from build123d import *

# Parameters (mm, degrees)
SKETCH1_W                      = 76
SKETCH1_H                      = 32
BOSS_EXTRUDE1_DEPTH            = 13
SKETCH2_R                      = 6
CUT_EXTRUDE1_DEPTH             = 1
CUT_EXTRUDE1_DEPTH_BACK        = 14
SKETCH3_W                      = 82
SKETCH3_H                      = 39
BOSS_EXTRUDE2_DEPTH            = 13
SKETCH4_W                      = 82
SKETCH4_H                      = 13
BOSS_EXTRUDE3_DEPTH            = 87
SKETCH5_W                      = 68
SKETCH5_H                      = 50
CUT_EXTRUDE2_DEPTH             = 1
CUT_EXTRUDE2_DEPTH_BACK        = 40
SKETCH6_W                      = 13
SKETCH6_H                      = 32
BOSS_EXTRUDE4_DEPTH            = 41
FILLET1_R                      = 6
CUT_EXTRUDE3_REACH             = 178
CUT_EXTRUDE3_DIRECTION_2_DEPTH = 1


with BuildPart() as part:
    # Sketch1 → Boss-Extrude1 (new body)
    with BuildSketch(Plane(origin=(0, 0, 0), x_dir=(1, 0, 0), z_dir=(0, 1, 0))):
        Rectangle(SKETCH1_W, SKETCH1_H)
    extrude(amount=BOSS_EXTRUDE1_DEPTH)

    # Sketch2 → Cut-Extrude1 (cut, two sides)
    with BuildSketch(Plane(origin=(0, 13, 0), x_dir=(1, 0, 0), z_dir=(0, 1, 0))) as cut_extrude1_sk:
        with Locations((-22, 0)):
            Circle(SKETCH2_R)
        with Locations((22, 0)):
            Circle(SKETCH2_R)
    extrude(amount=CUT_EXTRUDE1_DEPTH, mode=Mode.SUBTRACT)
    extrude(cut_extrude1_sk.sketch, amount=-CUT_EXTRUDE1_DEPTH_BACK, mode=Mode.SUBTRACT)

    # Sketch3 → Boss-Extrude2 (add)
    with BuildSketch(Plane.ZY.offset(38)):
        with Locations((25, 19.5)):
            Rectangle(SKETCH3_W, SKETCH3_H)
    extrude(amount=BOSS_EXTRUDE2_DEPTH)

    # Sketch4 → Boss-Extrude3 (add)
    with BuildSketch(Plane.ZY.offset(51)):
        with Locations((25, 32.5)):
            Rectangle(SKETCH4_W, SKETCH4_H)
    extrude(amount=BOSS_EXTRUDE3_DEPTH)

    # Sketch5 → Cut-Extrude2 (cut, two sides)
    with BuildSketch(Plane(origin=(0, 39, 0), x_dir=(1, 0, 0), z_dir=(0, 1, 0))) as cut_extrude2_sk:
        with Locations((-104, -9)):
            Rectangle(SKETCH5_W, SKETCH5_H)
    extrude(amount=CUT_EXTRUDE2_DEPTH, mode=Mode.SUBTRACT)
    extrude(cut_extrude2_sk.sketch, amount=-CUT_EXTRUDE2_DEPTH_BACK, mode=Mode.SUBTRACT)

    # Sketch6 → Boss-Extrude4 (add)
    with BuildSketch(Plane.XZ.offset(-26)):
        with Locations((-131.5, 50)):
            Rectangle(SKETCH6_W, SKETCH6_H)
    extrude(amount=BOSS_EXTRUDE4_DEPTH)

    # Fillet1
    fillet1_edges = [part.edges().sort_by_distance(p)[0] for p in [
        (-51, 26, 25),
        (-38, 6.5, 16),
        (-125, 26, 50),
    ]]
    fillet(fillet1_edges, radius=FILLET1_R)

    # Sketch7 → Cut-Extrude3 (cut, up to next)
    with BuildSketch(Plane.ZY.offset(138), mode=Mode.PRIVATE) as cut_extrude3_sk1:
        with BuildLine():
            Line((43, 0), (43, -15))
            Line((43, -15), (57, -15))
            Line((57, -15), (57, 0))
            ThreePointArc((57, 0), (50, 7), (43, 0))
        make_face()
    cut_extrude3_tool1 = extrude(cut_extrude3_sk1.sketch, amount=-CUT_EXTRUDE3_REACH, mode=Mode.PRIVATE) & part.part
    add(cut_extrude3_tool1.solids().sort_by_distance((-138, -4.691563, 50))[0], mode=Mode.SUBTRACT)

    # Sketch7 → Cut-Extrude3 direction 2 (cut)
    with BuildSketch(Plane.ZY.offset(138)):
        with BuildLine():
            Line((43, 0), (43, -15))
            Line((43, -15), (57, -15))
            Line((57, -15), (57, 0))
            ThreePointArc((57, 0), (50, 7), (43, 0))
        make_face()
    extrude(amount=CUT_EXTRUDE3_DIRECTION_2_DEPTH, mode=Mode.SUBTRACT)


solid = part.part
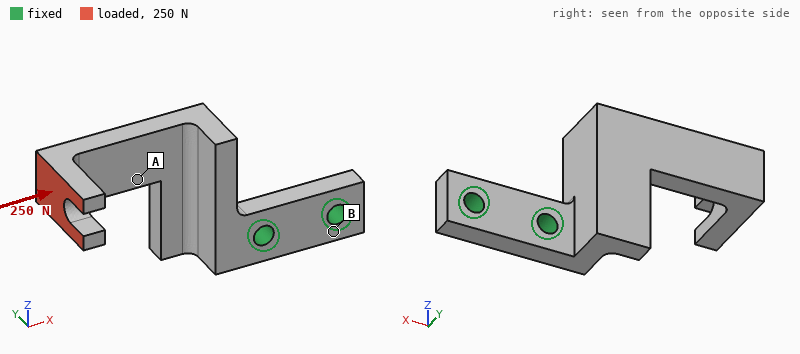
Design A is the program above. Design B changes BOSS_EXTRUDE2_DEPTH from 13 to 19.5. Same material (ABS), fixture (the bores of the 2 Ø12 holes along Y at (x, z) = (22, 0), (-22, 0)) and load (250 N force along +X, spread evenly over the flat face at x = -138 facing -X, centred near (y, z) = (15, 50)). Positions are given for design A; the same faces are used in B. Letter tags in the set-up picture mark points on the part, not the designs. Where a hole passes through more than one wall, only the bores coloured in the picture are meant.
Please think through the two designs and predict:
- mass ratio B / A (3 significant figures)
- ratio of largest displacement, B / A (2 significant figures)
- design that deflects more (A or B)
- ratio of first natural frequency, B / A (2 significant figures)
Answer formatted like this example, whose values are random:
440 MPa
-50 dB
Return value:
1.10
0.85
A
1.1
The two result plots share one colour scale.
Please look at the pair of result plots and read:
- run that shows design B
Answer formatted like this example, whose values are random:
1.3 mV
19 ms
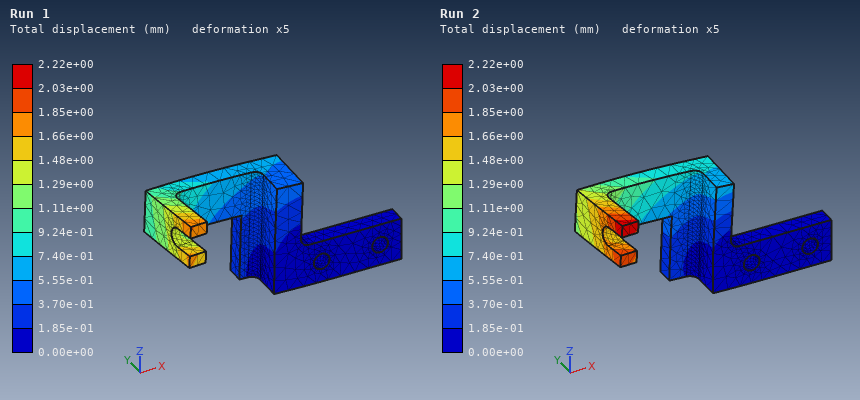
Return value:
Run 1
